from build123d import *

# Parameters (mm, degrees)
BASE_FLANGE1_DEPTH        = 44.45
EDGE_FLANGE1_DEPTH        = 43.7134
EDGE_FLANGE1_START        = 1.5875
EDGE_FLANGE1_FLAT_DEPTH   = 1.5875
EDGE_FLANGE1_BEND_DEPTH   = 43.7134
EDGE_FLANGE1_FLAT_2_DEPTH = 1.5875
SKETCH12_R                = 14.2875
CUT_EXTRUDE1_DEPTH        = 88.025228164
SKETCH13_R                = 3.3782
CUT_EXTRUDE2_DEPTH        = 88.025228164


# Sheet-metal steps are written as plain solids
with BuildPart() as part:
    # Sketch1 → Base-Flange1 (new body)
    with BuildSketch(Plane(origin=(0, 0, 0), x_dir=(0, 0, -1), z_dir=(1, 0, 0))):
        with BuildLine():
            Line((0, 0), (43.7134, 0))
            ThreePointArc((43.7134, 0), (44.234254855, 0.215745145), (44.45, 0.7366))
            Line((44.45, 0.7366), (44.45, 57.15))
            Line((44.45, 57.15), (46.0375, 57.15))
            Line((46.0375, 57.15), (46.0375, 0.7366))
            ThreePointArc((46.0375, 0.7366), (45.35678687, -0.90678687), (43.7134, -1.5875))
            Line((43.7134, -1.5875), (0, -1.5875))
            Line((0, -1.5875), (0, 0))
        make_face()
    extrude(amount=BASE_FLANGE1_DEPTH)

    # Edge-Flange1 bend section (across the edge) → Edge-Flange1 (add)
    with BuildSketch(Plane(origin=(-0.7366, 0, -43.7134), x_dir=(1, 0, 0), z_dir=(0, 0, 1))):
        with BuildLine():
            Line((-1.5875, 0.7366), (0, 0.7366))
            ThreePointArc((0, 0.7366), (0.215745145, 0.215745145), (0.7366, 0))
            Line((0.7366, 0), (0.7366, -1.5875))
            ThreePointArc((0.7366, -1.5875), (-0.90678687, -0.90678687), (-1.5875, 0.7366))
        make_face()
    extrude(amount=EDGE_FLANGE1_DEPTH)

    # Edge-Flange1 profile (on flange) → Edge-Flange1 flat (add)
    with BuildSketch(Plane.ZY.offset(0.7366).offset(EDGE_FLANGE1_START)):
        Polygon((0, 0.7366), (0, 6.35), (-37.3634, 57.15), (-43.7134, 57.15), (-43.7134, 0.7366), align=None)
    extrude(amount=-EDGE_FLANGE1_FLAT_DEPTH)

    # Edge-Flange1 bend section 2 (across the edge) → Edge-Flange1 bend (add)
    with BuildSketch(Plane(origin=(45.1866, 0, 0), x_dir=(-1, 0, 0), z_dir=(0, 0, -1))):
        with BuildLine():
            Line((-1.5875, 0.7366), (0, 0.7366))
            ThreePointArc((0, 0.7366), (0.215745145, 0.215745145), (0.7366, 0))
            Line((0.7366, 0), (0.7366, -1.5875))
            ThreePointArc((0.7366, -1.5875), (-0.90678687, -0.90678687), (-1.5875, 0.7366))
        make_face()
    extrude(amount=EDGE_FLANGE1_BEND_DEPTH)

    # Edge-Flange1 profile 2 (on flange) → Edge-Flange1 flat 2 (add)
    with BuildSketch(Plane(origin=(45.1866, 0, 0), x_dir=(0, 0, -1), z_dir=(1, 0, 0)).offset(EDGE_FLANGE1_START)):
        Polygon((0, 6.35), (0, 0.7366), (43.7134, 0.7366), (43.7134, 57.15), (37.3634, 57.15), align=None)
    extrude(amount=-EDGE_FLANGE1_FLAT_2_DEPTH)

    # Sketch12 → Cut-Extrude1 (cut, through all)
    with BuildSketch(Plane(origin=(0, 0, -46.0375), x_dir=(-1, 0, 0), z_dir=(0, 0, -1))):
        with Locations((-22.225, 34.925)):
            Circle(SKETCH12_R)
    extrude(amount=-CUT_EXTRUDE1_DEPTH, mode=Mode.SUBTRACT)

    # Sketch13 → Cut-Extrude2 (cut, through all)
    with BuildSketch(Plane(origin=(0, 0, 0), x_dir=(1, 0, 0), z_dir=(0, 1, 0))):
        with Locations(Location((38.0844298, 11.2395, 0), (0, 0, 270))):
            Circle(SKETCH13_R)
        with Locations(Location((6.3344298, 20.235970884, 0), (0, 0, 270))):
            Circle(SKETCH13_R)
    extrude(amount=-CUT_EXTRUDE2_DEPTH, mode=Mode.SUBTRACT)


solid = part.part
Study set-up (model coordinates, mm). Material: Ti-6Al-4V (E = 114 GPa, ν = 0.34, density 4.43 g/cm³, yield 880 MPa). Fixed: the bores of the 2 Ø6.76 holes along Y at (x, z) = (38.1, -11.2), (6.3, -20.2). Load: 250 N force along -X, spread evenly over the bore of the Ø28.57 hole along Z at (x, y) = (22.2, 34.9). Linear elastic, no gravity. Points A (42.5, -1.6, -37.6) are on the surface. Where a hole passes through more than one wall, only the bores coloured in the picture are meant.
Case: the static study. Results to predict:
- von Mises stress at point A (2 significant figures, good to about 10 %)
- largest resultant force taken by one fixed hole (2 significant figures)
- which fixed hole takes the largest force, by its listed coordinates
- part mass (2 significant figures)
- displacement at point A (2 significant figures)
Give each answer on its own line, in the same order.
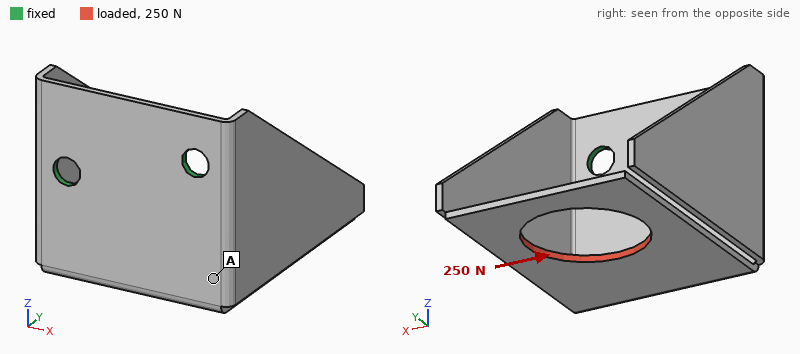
34 MPa
360 N
(6.3, -20.2)
50 g
0.30 mm
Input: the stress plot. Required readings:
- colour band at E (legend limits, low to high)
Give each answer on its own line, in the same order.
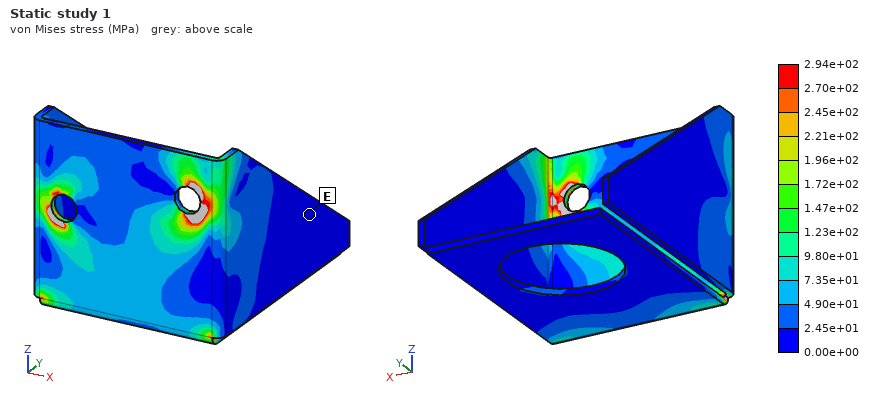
0.00e+00 to 2.45e+01 MPa
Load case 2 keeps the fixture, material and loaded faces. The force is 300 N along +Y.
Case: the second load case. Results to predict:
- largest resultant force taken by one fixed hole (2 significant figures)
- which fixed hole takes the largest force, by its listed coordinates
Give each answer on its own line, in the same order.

170 N
(6.3, -20.2)
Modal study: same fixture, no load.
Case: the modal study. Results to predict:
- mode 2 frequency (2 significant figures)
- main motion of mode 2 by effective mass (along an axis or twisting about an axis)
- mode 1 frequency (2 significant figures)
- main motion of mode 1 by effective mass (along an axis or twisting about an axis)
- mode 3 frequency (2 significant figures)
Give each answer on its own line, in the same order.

500 Hz
along X
340 Hz
along Z
520 Hz
